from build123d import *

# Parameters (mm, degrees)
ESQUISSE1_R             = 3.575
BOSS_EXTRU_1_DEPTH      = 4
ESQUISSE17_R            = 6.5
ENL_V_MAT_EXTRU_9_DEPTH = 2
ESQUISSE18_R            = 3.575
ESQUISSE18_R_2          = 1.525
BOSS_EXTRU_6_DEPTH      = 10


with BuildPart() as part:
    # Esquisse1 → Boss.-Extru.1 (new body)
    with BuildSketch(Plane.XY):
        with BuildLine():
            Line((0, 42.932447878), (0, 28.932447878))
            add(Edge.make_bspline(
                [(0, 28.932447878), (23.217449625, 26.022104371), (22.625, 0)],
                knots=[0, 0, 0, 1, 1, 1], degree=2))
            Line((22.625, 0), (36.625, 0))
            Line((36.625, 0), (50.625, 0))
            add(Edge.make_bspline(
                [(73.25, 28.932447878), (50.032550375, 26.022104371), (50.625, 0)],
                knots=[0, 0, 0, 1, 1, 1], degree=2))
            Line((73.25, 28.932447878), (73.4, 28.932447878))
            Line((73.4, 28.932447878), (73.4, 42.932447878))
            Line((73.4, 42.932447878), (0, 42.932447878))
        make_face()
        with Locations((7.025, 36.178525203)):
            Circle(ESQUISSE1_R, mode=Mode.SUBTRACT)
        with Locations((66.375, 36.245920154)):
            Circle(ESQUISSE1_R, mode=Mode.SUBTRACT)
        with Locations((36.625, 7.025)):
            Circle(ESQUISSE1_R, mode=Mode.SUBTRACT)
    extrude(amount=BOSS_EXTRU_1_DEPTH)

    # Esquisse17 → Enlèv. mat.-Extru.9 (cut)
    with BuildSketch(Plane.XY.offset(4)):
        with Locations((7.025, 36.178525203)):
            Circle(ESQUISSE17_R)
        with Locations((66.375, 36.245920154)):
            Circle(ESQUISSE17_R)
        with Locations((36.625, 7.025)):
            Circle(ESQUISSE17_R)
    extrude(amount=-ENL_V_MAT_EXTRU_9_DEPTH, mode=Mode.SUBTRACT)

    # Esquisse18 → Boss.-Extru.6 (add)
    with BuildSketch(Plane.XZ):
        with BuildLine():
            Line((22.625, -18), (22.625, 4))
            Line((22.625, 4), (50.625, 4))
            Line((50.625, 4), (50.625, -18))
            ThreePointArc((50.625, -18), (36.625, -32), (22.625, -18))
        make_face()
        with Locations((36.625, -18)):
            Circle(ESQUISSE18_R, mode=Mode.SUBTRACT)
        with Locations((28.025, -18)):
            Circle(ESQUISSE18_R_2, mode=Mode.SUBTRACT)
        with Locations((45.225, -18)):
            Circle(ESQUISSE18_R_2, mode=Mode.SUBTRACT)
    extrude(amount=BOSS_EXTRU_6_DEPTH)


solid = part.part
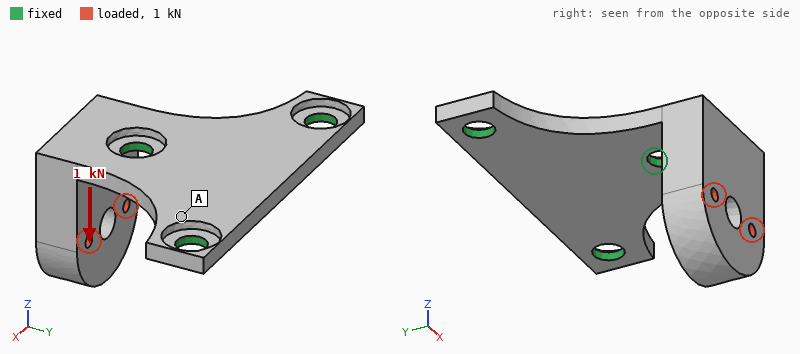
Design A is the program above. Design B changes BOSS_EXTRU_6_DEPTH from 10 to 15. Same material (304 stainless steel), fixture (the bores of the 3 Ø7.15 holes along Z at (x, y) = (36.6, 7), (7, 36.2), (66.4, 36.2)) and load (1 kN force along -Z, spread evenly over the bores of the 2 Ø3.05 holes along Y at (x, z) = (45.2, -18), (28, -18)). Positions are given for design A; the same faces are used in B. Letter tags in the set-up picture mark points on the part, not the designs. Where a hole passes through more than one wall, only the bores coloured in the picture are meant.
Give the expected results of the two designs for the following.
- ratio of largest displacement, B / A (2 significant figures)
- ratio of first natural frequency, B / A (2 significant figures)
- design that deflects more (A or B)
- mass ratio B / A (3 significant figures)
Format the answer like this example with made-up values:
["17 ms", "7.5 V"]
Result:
["1.4", "0.76", "B", "1.27"]
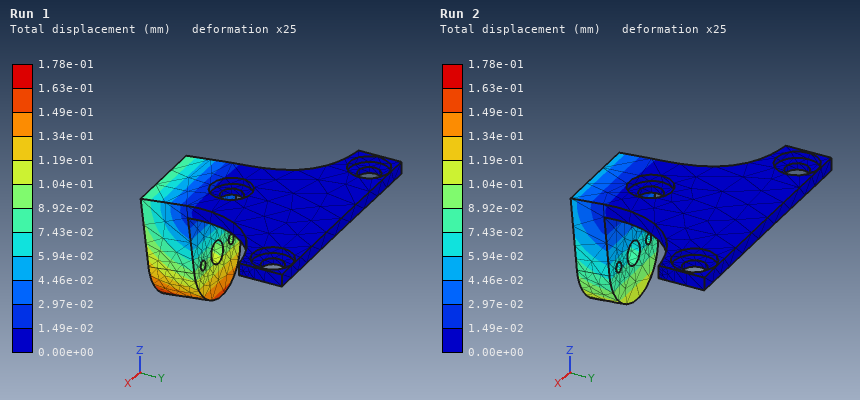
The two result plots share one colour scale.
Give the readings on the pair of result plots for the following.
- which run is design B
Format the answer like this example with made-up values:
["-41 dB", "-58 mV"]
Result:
["Run 1"]
